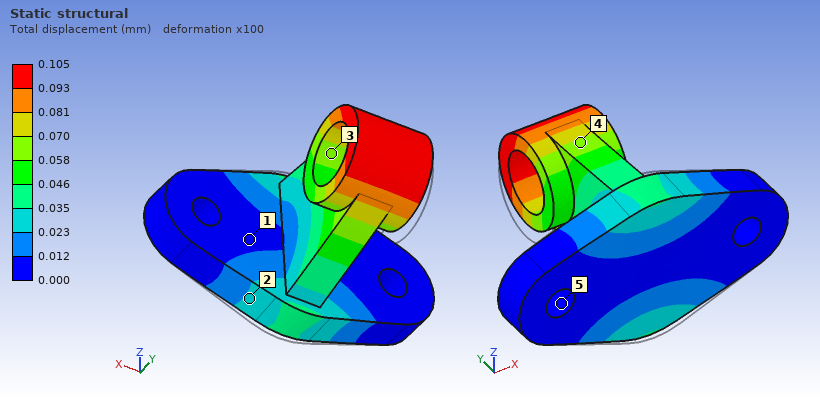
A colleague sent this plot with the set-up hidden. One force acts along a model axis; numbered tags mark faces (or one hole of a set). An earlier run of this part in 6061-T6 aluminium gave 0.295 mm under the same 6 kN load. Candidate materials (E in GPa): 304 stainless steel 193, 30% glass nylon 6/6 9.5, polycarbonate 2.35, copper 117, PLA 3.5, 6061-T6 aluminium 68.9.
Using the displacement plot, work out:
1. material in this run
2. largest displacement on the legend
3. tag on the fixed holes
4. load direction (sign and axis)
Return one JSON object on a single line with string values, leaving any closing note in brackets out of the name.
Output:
{"material in this run": "304 stainless steel", "largest displacement on the legend": "0.105 mm", "tag on the fixed holes": "5", "load direction": "+Z"}
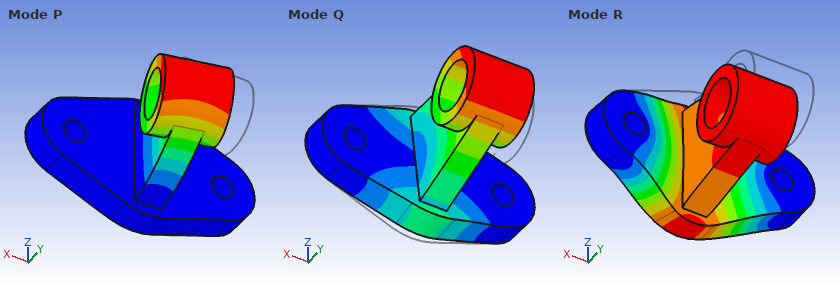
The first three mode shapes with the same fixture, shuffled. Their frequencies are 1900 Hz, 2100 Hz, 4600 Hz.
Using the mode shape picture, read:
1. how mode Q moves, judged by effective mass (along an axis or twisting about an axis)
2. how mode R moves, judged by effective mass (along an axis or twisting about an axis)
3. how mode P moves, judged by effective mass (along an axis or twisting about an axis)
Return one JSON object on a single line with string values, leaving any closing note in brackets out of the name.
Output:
{"how mode Q moves, judged by effective mass": "along Z", "how mode R moves, judged by effective mass": "along Y", "how mode P moves, judged by effective mass": "along X"}
